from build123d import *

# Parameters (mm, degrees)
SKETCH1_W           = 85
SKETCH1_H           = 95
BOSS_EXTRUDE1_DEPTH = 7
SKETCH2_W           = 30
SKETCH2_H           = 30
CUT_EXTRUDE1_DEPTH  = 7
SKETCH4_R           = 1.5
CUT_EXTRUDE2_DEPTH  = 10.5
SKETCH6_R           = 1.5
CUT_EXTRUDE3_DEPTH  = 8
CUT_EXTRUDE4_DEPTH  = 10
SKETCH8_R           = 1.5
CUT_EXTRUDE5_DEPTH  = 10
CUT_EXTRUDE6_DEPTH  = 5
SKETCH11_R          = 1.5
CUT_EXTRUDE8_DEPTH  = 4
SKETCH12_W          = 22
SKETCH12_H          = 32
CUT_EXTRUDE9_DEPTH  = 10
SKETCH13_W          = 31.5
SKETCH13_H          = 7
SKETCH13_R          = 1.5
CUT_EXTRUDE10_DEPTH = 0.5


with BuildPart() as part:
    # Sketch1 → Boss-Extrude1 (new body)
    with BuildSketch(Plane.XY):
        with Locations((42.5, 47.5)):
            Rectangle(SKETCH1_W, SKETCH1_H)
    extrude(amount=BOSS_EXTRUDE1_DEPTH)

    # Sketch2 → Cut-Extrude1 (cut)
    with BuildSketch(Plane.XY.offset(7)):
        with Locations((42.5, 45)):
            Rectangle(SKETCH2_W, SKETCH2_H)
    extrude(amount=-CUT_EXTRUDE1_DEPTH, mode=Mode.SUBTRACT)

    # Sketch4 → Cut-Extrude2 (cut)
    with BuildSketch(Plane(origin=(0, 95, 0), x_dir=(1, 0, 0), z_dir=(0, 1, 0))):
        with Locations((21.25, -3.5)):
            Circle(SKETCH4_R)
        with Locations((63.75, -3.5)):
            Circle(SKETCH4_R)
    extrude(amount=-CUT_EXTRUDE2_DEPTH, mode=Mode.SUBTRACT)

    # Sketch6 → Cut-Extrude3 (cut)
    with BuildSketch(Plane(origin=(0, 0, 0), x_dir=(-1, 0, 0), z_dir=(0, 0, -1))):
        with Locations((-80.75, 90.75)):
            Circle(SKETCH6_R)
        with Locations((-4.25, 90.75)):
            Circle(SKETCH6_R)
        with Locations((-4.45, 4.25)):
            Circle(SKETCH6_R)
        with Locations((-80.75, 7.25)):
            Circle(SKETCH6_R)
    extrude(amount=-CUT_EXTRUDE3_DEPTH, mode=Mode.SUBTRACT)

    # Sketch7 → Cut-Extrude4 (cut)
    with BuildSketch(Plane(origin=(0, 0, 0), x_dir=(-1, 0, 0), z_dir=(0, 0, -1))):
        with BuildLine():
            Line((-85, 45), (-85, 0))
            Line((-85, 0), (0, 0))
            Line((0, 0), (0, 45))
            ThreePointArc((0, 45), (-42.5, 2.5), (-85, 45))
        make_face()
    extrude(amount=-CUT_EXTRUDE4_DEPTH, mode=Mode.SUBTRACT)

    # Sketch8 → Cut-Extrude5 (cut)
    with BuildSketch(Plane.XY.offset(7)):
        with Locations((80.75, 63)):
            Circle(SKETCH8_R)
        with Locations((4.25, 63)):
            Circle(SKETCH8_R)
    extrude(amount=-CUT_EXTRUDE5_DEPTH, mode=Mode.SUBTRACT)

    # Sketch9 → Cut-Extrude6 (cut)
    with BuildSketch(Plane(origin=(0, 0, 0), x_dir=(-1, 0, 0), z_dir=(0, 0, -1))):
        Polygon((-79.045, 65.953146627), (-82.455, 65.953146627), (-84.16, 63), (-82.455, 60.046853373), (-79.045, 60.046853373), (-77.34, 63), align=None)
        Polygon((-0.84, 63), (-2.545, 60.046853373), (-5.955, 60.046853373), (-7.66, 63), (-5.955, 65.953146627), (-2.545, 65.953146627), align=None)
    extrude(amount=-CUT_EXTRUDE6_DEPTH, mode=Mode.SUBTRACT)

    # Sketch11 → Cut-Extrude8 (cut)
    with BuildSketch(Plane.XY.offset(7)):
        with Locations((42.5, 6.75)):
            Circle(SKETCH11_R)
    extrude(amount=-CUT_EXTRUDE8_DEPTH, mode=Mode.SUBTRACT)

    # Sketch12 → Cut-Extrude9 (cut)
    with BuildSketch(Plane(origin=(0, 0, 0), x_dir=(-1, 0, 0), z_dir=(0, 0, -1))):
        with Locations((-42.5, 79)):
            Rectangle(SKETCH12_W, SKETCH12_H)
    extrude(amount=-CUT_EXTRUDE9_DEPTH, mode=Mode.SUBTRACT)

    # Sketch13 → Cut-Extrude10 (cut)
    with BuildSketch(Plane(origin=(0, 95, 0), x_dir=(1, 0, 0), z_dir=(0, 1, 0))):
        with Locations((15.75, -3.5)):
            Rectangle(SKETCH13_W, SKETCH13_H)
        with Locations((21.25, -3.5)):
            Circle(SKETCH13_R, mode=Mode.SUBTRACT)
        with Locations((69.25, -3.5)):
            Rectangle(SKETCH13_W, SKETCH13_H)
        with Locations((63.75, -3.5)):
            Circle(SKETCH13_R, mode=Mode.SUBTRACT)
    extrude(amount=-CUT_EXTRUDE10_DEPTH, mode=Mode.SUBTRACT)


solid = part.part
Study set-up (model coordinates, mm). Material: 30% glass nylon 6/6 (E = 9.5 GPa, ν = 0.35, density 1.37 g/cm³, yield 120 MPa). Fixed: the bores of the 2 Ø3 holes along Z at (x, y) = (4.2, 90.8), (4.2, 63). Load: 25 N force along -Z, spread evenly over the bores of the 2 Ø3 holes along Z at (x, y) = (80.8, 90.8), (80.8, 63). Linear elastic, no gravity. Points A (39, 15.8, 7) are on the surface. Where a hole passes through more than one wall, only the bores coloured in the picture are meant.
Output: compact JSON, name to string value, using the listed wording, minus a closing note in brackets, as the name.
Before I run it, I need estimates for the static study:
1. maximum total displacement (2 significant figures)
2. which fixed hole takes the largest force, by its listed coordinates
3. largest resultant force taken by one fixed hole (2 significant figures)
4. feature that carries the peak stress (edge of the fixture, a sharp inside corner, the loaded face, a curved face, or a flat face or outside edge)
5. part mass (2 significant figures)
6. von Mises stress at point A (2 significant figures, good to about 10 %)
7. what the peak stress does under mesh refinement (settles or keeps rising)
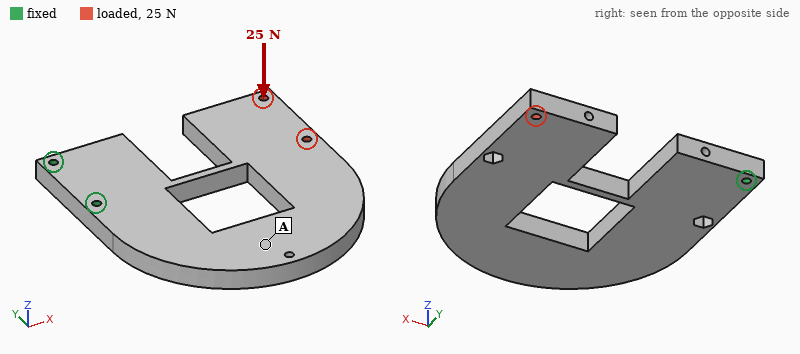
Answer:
{"maximum total displacement": "1.3 mm", "which fixed hole takes the largest force, by its listed coordinates": "(4.2, 90.8)", "largest resultant force taken by one fixed hole": "35 N", "feature that carries the peak stress": "edge of the fixture", "part mass": "51 g", "von Mises stress at point A": "3.4 MPa", "what the peak stress does under mesh refinement": "keeps rising"}
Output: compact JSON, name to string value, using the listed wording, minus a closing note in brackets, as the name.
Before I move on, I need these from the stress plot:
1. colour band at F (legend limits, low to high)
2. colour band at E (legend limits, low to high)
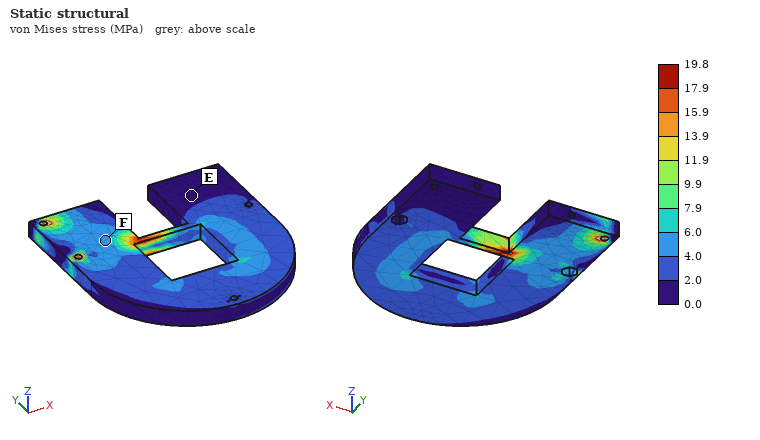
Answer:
{"colour band at F": "4.0 to 6.0 MPa", "colour band at E": "0.0 to 2.0 MPa"}
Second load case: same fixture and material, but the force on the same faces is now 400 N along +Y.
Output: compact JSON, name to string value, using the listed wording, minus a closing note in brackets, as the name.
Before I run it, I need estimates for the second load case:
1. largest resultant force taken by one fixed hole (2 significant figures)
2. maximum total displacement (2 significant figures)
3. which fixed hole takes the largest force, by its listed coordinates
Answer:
{"largest resultant force taken by one fixed hole": "1.2 kN", "maximum total displacement": "1.3 mm", "which fixed hole takes the largest force, by its listed coordinates": "(4.2, 90.8)"}
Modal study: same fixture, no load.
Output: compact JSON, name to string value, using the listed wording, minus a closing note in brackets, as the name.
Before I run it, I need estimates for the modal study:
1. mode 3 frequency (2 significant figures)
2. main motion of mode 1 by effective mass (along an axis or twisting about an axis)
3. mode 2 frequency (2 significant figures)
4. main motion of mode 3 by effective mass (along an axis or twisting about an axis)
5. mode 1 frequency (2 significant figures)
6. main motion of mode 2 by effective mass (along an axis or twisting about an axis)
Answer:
{"mode 3 frequency": "680 Hz", "main motion of mode 1 by effective mass": "along Z", "mode 2 frequency": "370 Hz", "main motion of mode 3 by effective mass": "along Y", "mode 1 frequency": "200 Hz", "main motion of mode 2 by effective mass": "twisting about X"}
